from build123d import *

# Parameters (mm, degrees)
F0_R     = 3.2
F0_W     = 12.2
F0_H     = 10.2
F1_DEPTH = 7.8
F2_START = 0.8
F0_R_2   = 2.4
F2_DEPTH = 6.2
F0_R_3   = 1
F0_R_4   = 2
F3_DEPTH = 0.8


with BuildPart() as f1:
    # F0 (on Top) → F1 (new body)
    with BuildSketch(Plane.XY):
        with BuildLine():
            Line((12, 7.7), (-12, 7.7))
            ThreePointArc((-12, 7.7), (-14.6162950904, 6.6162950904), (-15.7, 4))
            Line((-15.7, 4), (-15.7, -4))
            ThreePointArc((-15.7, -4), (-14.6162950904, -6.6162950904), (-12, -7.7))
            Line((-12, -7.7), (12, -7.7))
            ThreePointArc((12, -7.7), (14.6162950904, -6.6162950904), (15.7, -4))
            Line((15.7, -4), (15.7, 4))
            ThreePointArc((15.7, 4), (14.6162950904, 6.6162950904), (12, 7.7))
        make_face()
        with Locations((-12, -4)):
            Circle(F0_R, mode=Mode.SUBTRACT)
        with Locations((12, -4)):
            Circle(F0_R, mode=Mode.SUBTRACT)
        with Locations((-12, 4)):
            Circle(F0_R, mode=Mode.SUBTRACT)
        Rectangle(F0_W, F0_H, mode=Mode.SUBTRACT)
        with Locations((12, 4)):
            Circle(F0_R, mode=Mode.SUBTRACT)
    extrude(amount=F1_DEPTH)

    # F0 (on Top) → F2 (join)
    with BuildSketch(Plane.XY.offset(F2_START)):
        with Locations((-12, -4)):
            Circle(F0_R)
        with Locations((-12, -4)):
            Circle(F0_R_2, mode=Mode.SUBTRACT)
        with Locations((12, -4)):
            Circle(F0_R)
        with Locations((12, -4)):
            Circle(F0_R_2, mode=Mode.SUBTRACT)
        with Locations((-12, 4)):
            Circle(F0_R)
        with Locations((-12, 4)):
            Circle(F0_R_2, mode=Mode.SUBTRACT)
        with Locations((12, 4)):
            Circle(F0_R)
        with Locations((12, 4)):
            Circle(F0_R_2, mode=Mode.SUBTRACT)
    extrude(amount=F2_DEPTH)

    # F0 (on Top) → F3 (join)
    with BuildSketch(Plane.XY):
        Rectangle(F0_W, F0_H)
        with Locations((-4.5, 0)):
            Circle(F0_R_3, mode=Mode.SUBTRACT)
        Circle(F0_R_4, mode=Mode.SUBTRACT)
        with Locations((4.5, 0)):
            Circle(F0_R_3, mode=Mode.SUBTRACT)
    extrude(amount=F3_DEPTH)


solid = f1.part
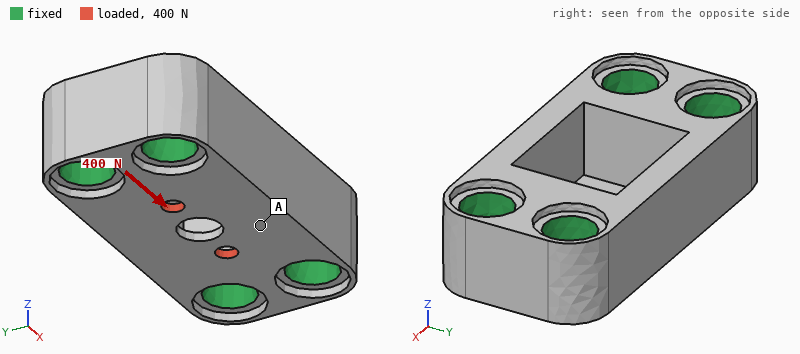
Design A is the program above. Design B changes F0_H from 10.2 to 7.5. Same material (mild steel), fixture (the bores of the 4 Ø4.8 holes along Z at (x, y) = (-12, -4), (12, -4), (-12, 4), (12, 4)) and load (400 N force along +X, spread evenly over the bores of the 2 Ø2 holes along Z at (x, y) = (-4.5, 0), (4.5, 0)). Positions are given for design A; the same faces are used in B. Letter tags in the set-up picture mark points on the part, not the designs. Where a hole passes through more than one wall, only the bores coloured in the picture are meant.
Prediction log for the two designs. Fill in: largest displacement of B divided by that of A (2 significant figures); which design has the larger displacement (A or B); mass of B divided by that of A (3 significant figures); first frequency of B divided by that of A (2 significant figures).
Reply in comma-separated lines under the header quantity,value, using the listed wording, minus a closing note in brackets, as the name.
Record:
quantity,value
largest displacement of B divided by that of A,0.92
which design has the larger displacement,A
mass of B divided by that of A,1.11
first frequency of B divided by that of A,1.1
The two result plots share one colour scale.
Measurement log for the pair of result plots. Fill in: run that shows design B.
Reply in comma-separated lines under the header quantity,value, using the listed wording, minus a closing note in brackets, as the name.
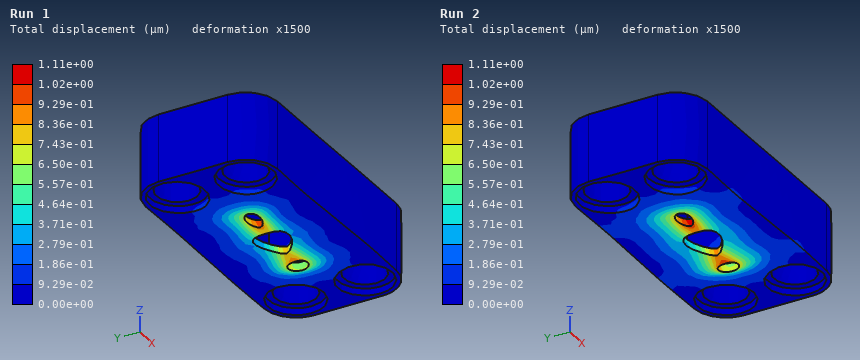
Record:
quantity,value
run that shows design B,Run 1
